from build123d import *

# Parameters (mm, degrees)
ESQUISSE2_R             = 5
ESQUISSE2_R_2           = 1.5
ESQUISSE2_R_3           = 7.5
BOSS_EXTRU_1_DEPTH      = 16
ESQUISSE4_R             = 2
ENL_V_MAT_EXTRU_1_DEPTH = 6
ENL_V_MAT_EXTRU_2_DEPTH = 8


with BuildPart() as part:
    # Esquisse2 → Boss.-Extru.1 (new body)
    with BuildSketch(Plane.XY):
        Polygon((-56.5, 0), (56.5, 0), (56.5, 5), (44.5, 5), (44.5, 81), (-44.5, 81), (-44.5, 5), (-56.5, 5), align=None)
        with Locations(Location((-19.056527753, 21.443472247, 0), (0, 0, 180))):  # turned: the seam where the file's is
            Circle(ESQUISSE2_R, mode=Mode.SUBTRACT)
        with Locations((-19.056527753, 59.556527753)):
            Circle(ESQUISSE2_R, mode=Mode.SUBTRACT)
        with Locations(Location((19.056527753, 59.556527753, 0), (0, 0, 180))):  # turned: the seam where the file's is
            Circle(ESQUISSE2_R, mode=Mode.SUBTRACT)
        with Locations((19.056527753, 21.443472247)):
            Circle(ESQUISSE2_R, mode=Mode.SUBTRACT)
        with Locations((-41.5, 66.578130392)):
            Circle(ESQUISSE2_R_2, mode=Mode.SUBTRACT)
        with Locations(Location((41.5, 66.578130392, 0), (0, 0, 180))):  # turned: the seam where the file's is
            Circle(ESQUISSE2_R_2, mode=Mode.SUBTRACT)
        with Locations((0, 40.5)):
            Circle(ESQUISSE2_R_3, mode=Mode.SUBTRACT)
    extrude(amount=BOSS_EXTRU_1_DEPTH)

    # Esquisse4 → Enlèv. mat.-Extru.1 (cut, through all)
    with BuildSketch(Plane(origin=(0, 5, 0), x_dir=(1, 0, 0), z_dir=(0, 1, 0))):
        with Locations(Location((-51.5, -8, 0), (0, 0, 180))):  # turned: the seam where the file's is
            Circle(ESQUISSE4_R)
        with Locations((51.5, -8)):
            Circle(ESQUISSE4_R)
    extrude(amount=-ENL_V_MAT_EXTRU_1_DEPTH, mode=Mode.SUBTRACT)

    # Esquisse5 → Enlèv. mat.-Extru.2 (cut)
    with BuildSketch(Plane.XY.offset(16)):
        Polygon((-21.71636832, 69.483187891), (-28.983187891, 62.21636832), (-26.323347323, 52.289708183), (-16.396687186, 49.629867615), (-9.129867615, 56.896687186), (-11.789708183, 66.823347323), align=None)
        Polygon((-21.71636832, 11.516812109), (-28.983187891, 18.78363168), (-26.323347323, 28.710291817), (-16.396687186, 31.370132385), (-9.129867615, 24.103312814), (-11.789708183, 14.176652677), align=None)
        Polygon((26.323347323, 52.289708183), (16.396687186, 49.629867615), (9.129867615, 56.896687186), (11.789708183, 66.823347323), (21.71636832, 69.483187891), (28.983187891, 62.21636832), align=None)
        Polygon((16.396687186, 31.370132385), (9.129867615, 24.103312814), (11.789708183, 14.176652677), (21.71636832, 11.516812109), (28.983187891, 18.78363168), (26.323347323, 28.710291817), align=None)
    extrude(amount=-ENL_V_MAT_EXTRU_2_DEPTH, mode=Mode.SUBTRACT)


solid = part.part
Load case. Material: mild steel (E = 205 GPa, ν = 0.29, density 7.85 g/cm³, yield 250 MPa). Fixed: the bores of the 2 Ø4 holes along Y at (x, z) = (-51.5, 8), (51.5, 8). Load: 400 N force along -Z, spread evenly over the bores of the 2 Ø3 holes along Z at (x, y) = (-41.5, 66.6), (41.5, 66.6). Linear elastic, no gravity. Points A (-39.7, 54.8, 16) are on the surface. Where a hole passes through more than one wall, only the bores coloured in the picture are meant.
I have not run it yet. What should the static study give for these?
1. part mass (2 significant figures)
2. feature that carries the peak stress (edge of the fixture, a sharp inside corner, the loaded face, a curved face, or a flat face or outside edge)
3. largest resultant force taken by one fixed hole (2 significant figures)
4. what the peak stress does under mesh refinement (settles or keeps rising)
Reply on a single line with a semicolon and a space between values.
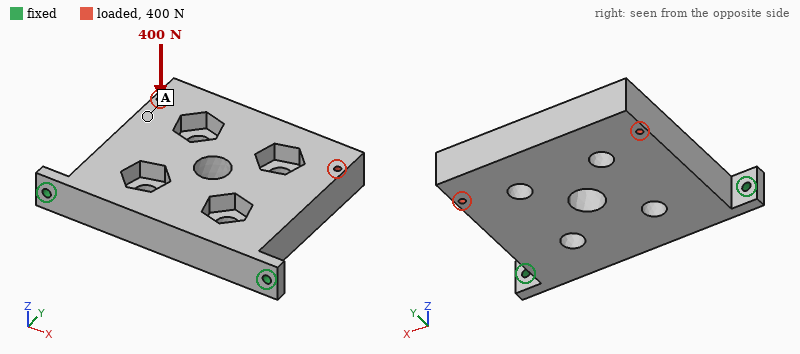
810 g; edge of the fixture; 200 N; keeps rising
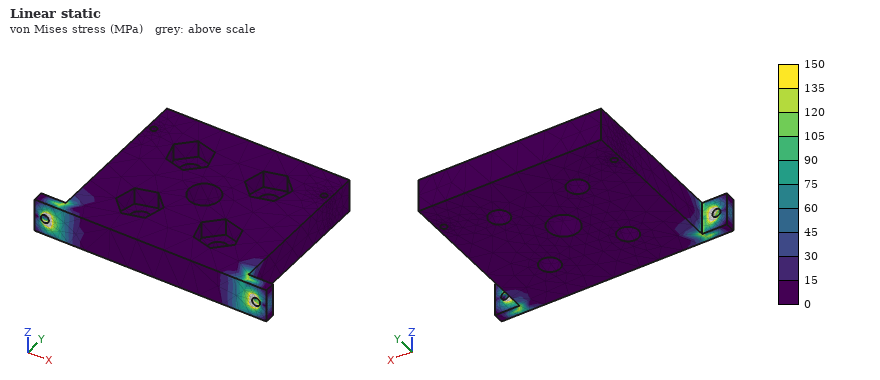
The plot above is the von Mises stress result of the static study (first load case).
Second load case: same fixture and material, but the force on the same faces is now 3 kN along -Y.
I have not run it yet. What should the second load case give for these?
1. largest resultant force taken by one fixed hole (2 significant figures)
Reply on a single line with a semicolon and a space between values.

1.7 kN
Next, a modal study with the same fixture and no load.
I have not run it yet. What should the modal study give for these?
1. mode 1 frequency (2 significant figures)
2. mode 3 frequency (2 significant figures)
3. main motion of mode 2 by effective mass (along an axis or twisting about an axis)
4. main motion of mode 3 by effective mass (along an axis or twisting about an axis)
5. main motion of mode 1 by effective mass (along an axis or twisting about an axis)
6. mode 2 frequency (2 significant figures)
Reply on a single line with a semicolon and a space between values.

420 Hz; 3200 Hz; twisting about Y; along X; along Z; 2900 Hz
